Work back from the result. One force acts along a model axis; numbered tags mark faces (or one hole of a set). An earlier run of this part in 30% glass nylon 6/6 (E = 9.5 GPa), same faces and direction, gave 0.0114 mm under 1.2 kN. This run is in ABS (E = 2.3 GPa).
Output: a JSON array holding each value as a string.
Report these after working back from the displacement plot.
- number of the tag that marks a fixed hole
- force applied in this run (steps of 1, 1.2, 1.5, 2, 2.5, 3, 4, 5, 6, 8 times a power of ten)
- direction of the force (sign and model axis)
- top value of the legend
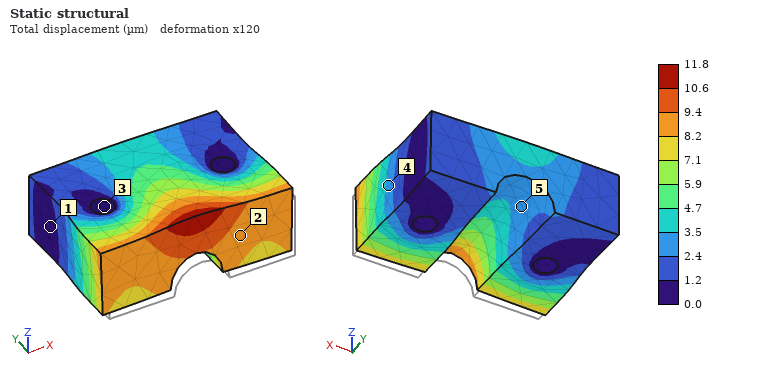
["3", "300 N", "+Y", "11.8 µm"]
